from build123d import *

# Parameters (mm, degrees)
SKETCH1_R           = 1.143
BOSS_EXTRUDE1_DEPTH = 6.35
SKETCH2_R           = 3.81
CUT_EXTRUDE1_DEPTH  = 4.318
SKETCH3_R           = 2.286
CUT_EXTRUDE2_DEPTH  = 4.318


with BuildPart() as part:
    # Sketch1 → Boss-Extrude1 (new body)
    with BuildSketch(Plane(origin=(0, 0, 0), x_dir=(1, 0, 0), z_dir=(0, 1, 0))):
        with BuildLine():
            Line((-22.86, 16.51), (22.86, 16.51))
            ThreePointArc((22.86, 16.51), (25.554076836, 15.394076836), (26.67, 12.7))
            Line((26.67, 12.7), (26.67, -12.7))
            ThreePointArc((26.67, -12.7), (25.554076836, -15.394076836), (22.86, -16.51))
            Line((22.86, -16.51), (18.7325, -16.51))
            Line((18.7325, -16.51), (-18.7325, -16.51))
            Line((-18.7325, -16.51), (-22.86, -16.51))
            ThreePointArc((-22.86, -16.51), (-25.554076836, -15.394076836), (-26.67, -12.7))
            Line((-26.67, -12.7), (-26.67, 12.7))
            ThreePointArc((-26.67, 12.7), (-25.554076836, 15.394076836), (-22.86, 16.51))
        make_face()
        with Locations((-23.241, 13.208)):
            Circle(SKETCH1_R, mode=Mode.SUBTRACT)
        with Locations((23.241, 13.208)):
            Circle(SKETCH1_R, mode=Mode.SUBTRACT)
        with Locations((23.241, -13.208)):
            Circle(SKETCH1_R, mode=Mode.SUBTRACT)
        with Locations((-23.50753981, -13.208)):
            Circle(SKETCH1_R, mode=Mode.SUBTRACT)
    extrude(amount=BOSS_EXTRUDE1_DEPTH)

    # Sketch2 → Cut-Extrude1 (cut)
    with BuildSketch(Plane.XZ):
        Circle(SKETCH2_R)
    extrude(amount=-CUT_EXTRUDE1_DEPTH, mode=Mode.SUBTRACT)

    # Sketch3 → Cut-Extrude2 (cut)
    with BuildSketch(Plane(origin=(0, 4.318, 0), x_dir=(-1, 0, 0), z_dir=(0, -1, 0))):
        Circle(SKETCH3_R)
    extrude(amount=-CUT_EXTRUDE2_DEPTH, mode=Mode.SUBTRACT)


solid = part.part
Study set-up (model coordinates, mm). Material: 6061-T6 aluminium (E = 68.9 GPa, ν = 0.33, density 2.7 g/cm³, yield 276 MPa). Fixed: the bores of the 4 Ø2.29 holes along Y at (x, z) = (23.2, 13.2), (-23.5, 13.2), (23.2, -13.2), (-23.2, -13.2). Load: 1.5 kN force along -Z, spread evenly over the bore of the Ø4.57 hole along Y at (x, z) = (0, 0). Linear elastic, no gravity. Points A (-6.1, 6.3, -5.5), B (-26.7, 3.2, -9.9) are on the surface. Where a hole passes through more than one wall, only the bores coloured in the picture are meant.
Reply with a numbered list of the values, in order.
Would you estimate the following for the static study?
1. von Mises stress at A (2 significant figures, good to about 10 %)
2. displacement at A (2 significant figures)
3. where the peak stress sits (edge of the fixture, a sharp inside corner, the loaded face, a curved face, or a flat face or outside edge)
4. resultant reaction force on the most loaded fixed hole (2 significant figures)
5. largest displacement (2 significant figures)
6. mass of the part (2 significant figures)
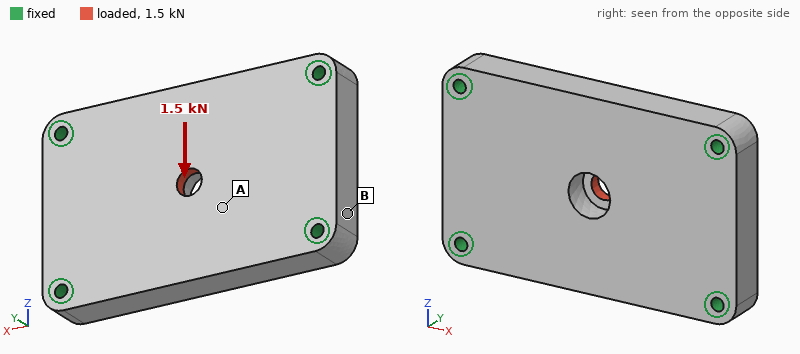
1. 16 MPa
2. 4.5 µm
3. a sharp inside corner
4. 500 N
5. 8.0 µm
6. 29 g
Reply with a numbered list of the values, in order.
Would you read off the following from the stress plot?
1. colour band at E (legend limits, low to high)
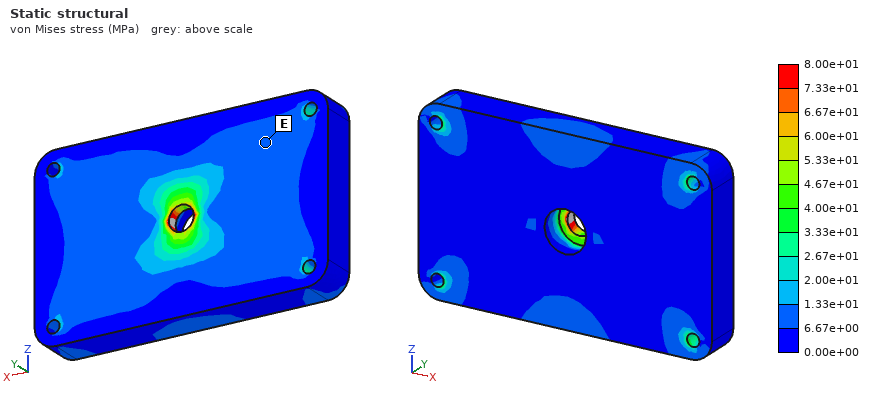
1. 6.67e+00 to 1.33e+01 MPa
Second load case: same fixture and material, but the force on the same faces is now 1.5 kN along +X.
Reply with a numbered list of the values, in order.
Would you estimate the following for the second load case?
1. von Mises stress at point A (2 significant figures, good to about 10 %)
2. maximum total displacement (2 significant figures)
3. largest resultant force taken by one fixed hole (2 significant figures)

1. 13 MPa
2. 5.5 µm
3. 400 N
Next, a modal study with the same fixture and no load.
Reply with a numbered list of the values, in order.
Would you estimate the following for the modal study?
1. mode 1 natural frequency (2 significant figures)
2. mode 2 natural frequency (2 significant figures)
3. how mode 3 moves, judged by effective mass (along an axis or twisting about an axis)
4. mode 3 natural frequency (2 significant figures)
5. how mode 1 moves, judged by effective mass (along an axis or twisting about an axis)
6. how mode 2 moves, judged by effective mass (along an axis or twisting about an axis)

1. 11 kHz
2. 17 kHz
3. twisting about Z
4. 27 kHz
5. along Y
6. twisting about X
